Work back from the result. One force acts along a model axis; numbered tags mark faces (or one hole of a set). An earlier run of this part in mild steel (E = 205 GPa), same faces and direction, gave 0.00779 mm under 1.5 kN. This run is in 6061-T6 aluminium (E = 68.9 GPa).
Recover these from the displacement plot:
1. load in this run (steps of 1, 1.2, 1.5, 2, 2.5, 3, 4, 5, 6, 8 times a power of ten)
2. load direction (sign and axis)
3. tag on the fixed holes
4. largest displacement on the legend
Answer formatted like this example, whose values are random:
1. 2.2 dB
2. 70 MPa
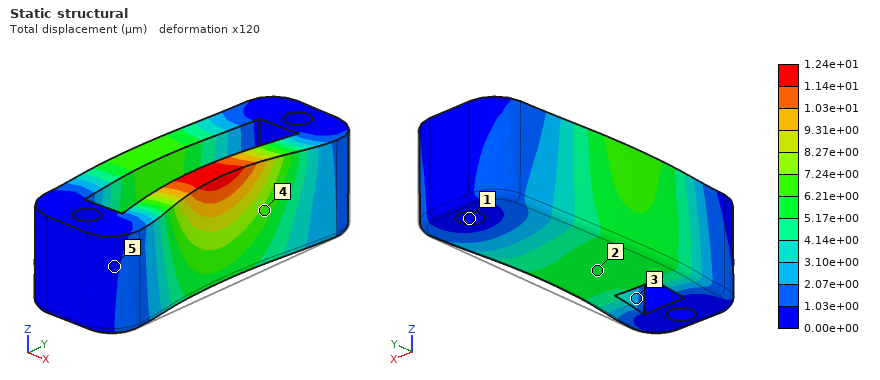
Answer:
1. 800 N
2. -X
3. 1
4. 1.24e+01 µm
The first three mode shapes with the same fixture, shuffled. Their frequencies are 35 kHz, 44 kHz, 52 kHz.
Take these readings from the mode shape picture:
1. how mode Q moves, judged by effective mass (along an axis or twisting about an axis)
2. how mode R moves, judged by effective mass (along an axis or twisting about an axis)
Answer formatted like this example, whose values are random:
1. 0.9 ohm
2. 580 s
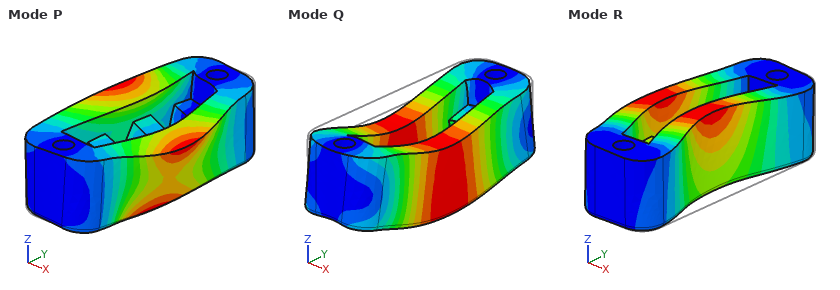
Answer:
1. along Z
2. along X
